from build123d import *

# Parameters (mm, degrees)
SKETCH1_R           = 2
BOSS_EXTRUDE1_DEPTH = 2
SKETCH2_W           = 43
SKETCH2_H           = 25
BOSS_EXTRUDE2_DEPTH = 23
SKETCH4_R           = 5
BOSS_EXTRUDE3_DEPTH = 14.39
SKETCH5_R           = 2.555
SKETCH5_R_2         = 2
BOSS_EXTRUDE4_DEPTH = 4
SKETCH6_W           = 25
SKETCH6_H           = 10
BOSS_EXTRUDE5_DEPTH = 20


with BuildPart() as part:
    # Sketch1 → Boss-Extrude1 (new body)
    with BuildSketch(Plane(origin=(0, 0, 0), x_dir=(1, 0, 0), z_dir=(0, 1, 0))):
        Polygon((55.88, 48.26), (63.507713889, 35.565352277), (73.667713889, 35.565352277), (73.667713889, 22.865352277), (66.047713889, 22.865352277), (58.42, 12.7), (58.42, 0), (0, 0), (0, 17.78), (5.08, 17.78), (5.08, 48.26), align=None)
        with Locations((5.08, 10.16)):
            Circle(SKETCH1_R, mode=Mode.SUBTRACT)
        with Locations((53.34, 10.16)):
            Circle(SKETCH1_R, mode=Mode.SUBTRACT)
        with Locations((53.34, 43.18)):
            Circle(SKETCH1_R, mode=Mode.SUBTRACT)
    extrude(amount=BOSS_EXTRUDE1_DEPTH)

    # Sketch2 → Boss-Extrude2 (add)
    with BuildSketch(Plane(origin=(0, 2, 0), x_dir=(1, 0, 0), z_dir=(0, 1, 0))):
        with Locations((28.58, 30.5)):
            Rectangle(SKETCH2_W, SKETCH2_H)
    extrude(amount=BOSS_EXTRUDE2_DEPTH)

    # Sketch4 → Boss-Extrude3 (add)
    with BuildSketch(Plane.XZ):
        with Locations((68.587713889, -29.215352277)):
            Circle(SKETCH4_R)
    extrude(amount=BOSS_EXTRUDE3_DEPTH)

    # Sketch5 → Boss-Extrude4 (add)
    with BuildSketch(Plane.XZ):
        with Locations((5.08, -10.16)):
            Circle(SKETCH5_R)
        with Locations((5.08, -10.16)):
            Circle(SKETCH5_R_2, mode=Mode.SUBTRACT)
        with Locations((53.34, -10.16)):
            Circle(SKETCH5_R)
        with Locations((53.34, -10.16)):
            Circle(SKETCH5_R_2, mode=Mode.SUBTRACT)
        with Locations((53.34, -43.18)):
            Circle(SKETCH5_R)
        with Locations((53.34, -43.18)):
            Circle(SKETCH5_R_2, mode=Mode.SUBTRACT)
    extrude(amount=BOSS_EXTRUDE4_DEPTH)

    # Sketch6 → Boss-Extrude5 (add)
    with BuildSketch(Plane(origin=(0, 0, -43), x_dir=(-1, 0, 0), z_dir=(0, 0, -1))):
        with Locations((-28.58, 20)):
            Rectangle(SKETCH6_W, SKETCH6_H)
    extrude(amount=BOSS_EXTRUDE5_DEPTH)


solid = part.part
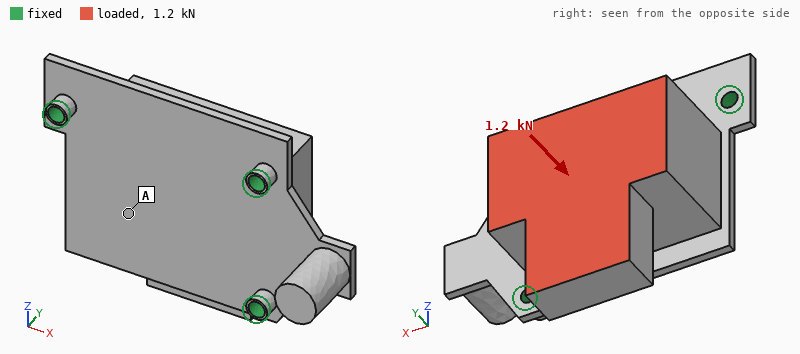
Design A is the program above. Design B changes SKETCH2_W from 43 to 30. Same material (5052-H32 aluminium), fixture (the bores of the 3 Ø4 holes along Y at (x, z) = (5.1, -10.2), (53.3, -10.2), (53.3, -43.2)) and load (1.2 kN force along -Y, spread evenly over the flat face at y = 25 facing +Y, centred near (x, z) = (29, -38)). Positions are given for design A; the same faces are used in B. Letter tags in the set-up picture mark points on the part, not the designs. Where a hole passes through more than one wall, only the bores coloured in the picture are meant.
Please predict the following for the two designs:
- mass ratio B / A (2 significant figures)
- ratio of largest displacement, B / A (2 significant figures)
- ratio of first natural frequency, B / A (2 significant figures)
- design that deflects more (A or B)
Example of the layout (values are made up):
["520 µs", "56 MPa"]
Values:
["0.80", "3.3", "0.67", "B"]
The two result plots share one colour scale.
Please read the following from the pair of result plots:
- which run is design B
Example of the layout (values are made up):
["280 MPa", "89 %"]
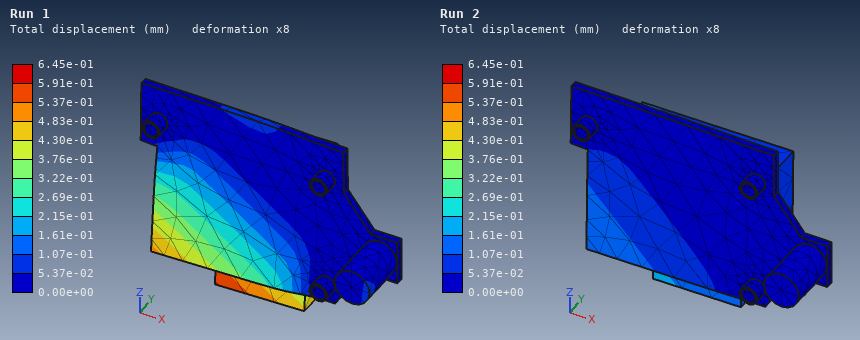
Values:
["Run 1"]
